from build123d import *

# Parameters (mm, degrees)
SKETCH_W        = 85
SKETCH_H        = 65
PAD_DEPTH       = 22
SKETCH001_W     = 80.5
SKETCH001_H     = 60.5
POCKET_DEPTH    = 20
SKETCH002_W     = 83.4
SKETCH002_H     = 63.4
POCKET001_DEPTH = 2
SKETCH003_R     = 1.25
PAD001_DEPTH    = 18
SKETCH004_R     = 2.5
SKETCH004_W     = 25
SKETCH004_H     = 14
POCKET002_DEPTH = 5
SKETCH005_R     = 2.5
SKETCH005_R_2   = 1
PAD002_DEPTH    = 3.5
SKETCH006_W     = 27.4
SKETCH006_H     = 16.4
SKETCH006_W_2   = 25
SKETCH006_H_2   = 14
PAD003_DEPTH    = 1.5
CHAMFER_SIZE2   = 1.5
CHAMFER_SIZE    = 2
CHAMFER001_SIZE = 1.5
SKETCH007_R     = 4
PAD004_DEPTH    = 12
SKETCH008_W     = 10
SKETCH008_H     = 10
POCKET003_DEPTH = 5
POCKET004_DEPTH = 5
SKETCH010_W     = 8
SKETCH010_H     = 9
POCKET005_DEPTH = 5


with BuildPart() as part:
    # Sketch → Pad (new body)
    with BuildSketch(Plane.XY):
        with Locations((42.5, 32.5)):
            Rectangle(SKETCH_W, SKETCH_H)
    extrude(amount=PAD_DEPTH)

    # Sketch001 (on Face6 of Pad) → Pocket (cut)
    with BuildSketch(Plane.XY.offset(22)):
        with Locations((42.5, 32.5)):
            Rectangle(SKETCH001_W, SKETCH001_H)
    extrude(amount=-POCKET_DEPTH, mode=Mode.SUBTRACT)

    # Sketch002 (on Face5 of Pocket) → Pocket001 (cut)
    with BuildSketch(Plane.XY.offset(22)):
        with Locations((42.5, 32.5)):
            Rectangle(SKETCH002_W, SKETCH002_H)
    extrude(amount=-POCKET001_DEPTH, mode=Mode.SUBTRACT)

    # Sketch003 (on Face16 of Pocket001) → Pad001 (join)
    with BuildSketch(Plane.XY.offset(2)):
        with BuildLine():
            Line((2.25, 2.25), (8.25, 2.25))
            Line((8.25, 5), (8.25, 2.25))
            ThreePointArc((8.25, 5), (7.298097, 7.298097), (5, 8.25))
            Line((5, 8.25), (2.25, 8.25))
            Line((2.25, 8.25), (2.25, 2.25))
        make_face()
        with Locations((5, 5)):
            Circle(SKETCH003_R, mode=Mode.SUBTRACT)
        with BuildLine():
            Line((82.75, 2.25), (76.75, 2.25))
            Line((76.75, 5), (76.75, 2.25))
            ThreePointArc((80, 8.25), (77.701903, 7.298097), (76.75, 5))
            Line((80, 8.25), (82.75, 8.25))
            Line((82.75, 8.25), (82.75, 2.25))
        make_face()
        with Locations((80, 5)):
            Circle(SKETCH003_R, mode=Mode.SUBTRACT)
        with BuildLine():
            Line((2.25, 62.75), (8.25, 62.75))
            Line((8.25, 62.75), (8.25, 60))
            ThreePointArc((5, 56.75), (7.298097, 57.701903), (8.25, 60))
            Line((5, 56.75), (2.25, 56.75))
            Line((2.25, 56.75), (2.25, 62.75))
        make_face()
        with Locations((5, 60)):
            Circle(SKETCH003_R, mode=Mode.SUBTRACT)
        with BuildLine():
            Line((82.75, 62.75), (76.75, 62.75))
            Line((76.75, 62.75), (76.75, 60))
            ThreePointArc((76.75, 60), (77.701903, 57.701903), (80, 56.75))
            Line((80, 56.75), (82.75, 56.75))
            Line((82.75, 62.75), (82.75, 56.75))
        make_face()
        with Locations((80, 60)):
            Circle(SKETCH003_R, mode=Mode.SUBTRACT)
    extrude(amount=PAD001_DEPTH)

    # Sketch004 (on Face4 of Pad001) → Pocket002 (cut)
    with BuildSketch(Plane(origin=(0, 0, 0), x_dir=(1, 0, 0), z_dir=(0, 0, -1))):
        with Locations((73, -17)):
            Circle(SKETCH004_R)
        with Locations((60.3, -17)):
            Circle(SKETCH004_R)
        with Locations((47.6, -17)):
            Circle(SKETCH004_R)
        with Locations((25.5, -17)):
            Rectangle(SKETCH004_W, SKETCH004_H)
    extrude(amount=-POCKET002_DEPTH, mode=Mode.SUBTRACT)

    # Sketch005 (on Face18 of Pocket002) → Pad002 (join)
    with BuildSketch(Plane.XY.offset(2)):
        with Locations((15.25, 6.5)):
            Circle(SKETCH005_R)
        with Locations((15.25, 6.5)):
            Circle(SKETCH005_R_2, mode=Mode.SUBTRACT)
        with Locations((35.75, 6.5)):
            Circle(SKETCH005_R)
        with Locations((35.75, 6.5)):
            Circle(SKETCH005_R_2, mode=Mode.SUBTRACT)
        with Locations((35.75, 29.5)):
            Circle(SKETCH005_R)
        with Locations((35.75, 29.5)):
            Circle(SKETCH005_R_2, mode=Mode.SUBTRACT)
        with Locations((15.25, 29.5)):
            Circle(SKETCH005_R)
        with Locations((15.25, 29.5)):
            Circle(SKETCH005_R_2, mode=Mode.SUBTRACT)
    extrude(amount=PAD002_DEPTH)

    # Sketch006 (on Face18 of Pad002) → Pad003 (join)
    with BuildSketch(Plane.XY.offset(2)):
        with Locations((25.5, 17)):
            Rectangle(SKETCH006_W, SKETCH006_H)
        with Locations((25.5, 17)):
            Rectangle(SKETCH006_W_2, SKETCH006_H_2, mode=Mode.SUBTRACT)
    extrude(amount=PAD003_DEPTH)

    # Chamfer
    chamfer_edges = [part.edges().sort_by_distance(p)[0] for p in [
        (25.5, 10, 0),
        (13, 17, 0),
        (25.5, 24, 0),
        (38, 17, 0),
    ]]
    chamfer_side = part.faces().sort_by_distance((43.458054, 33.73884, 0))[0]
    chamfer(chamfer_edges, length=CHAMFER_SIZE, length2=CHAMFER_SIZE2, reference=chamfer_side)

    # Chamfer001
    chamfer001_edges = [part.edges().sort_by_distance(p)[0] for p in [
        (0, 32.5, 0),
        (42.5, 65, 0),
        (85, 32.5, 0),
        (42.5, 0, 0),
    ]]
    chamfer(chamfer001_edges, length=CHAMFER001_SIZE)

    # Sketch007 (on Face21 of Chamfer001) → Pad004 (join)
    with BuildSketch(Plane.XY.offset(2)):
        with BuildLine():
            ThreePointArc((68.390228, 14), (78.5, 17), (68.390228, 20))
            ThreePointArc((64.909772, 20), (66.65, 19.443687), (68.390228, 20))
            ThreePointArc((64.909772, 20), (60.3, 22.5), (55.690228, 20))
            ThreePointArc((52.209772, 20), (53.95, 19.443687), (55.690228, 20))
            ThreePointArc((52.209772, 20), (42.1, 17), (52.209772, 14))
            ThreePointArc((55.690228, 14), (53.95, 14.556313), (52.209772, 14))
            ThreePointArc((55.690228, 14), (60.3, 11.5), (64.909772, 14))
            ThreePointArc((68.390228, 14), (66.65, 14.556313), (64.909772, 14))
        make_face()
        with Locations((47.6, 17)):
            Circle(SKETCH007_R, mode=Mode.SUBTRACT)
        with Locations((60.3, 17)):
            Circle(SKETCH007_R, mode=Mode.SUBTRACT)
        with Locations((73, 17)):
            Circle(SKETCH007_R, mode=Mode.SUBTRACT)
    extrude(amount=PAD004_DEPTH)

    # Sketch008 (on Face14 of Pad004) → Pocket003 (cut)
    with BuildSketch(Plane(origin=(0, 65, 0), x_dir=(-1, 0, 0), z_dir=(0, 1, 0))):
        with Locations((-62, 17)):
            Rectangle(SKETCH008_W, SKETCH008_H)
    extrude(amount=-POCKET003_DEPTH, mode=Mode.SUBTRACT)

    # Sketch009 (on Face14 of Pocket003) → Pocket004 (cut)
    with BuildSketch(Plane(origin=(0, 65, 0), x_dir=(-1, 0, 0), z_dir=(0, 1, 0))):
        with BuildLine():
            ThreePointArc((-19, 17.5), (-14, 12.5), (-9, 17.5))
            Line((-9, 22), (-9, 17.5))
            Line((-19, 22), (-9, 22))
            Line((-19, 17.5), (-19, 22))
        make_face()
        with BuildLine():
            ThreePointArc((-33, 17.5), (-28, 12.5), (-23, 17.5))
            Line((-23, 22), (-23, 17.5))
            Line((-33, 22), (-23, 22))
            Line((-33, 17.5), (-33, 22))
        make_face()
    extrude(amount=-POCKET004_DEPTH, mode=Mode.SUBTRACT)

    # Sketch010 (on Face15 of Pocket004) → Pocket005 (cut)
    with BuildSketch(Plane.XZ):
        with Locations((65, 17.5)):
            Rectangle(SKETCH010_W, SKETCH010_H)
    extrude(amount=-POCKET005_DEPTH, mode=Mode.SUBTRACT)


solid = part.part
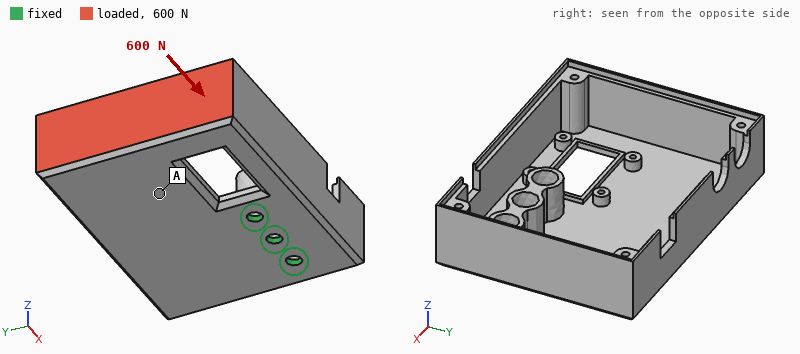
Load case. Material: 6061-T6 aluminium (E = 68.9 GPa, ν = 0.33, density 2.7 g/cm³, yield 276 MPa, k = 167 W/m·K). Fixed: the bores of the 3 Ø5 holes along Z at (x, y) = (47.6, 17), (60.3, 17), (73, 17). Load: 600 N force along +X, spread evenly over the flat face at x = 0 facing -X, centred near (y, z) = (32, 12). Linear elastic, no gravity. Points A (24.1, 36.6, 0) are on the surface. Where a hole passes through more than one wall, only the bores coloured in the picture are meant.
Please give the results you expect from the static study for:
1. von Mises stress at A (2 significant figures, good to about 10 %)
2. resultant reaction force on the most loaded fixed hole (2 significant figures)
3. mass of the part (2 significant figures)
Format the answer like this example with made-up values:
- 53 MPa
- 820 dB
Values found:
- 7.5 MPa
- 430 N
- 69 g
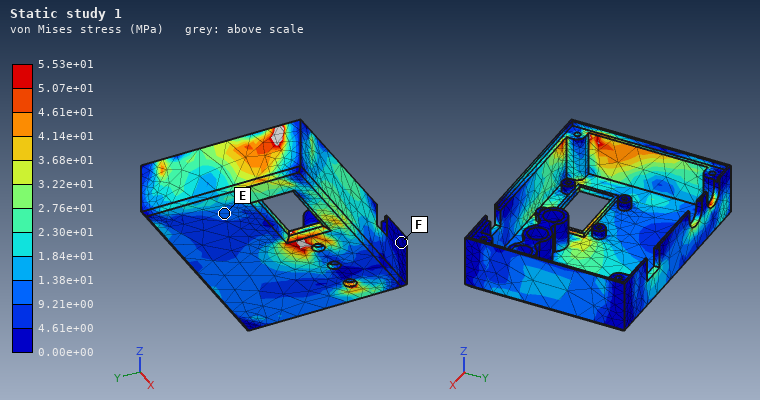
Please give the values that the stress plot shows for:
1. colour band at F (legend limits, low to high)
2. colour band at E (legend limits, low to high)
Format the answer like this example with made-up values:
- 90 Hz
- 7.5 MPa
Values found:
- 0.00e+00 to 4.61e+00 MPa
- 9.21e+00 to 1.38e+01 MPa
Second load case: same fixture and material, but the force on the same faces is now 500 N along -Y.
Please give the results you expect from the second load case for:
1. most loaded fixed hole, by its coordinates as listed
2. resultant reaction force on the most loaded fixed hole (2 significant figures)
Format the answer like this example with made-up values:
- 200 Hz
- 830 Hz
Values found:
- (47.6, 17)
- 1.3 kN
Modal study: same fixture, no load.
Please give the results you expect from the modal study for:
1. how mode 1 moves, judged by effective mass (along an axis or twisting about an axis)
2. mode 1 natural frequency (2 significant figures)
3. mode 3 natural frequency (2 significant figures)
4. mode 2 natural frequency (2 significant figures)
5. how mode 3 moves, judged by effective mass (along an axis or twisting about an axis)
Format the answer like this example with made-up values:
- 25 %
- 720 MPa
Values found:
- along Z
- 440 Hz
- 1100 Hz
- 1000 Hz
- along Z
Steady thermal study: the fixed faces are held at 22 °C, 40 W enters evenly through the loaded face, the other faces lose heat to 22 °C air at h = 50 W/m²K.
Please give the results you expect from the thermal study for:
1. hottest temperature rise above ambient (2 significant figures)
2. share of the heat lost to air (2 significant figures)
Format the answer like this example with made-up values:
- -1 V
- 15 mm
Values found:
- 64 K
- 58 %
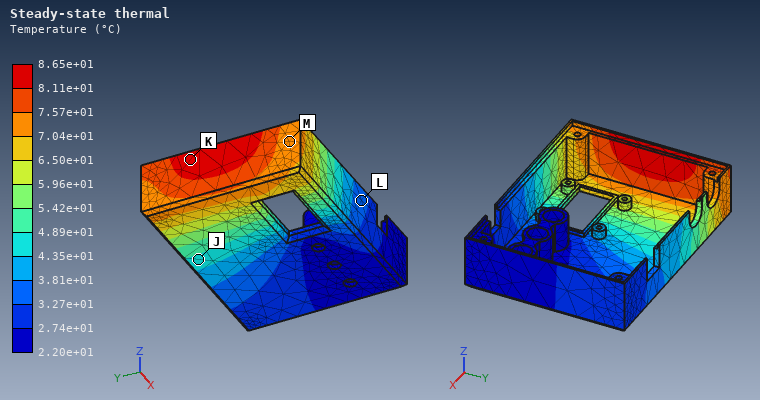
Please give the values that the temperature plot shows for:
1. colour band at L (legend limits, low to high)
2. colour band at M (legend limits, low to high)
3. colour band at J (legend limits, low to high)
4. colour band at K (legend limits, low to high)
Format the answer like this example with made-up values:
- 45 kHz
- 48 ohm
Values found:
- 3.27e+01 to 3.81e+01 °C
- 7.04e+01 to 7.57e+01 °C
- 4.35e+01 to 4.89e+01 °C
- 8.11e+01 to 8.65e+01 °C
